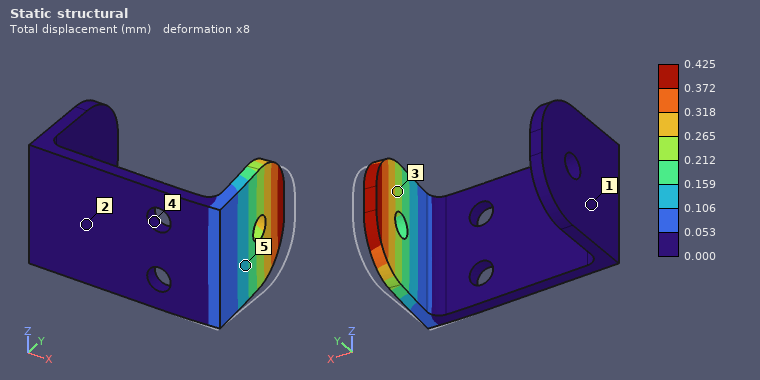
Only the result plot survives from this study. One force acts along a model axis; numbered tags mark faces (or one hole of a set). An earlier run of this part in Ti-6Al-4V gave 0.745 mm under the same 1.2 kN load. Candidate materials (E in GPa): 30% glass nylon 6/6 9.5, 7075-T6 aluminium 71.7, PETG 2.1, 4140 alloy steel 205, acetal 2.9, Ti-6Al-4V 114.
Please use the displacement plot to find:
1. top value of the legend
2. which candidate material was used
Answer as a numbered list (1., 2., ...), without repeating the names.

1. 0.425 mm
2. 4140 alloy steel
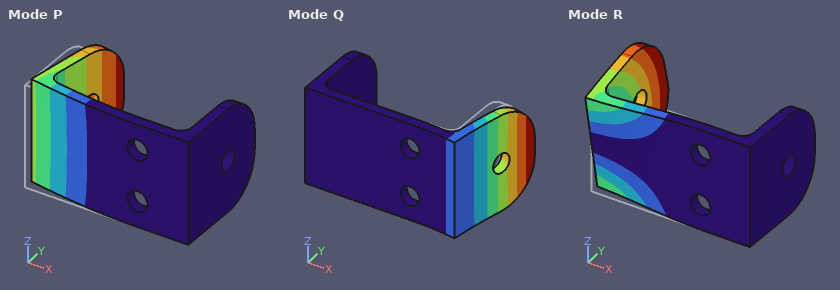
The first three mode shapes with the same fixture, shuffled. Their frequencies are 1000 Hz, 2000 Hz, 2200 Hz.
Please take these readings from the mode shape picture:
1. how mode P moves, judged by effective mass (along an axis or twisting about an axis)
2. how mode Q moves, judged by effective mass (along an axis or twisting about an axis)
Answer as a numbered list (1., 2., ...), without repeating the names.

1. along Y
2. along X
